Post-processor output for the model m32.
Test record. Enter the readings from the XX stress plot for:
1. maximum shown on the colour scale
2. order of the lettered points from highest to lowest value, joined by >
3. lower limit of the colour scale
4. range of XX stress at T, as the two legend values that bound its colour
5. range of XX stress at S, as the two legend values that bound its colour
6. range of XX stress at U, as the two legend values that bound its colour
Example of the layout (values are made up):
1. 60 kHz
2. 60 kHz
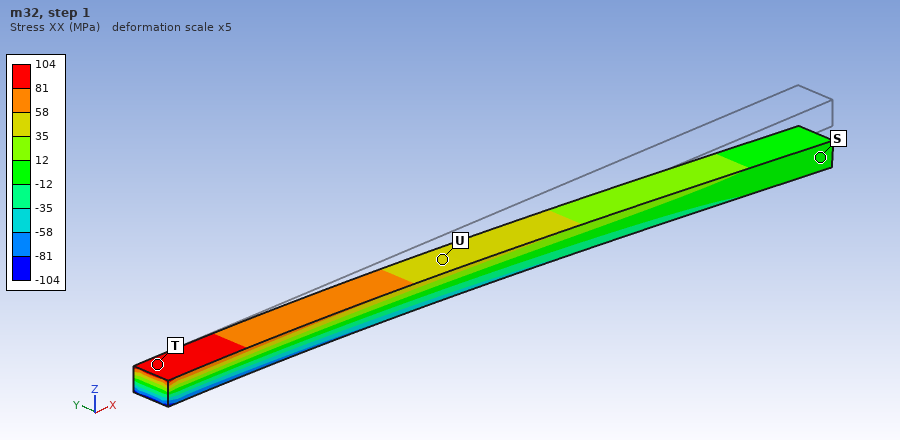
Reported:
1. 104 MPa
2. T > U > S
3. -104 MPa
4. 81 to 104 MPa
5. -12 to 12 MPa
6. 35 to 58 MPa
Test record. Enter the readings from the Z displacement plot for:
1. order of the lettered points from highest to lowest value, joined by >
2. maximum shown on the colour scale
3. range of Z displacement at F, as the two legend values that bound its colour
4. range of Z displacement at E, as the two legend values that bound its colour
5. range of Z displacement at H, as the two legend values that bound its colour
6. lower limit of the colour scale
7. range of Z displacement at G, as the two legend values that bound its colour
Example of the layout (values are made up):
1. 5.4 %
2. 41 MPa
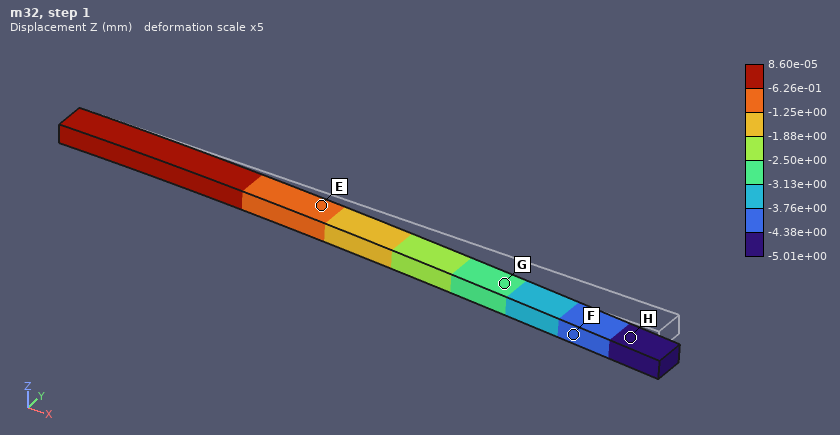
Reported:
1. E > G > F > H
2. 8.60e-05 mm
3. -4.38e+00 to -3.76e+00 mm
4. -1.25e+00 to -6.26e-01 mm
5. -5.01e+00 to -4.38e+00 mm
6. -5.01e+00 mm
7. -3.13e+00 to -2.50e+00 mm
